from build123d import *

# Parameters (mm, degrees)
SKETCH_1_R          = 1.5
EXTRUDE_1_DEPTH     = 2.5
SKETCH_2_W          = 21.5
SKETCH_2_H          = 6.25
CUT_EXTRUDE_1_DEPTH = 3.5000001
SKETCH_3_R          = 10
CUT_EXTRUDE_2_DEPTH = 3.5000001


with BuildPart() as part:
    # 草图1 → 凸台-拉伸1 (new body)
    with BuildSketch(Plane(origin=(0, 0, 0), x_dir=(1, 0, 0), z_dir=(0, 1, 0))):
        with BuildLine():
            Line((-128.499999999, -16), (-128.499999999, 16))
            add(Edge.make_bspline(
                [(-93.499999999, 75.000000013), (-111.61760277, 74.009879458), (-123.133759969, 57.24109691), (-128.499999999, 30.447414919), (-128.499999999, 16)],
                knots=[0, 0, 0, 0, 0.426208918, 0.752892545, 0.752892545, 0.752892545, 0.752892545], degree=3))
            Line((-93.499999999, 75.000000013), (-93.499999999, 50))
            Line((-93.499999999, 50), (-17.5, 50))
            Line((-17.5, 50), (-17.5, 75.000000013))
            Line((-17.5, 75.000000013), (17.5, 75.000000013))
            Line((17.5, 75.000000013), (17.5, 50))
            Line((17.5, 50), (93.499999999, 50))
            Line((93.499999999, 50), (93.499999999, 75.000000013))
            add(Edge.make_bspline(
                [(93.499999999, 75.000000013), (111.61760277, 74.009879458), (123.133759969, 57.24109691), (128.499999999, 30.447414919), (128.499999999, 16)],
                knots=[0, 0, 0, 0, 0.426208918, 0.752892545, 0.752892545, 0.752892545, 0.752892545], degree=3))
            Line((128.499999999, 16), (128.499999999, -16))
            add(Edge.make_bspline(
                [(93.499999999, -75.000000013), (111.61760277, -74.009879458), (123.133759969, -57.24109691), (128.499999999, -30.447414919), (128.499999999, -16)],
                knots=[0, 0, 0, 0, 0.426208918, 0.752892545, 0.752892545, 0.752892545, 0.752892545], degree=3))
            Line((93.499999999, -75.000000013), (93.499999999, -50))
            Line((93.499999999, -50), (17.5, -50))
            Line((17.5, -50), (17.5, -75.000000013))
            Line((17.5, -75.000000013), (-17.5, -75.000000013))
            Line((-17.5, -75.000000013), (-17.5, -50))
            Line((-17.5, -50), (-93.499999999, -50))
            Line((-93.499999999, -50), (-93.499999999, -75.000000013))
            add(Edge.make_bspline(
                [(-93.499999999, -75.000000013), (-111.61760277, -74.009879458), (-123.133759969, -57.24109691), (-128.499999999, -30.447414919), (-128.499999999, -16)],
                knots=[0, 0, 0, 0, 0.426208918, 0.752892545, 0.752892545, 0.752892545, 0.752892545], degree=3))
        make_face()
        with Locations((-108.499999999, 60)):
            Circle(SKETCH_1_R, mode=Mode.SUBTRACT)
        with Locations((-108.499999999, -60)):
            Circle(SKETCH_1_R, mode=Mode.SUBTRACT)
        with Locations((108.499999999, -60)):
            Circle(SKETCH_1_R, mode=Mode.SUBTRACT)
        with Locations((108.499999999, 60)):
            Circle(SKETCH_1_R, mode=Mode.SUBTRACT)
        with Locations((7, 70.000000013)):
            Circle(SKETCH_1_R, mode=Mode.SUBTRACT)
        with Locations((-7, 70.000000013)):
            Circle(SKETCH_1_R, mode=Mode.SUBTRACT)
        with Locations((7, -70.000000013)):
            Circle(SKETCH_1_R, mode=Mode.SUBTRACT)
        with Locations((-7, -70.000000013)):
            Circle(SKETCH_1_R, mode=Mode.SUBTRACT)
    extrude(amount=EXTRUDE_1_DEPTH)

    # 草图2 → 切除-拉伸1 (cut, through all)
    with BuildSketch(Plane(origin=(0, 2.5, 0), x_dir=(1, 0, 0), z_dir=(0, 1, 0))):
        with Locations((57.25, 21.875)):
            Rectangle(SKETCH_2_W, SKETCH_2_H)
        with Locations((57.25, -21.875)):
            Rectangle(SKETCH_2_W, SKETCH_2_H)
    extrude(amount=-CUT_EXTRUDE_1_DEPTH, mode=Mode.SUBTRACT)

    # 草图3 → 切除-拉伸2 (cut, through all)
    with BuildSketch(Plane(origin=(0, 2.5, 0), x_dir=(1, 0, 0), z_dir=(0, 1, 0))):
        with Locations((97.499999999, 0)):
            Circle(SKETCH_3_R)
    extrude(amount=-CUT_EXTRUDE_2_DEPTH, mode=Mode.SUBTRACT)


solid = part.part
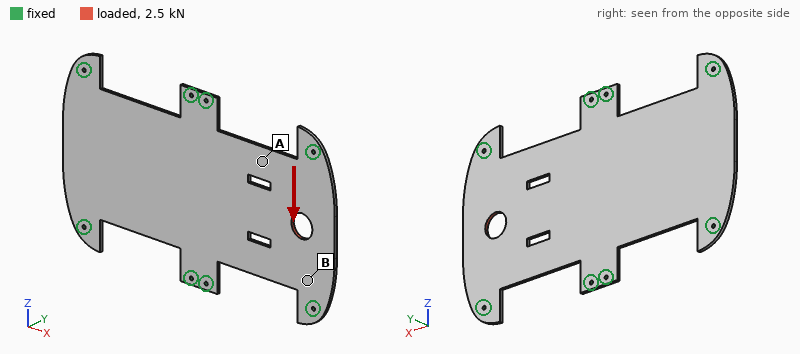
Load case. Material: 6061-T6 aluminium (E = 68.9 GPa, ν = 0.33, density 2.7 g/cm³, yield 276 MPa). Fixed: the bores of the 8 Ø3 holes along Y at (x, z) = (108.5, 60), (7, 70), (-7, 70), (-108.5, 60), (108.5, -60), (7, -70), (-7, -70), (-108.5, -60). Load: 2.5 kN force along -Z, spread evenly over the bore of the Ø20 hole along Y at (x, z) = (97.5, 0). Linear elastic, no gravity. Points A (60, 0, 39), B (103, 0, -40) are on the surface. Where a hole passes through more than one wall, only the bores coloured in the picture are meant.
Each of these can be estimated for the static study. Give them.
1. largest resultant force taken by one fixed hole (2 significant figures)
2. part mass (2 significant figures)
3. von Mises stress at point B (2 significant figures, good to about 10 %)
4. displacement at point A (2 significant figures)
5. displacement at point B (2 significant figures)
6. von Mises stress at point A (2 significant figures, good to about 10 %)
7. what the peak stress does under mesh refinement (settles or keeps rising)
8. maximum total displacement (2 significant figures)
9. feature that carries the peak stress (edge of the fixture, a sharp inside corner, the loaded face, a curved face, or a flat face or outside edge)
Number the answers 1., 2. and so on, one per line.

1. 1.1 kN
2. 190 g
3. 16 MPa
4. 8.4 µm
5. 7.2 µm
6. 3.9 MPa
7. keeps rising
8. 15 µm
9. edge of the fixture
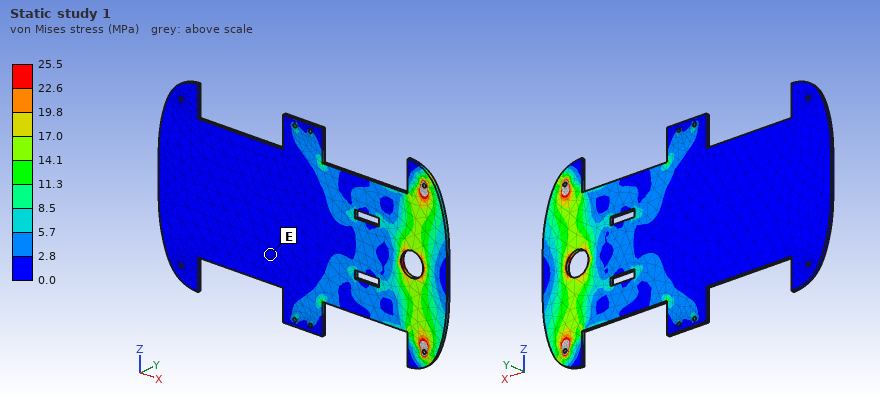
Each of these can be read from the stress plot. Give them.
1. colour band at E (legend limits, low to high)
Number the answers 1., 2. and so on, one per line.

1. 0.0 to 2.8 MPa
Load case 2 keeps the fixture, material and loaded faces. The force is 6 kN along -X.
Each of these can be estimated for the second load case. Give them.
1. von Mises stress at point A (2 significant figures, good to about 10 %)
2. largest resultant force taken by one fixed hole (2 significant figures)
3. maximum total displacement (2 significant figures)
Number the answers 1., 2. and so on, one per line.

1. 16 MPa
2. 1.3 kN
3. 74 µm
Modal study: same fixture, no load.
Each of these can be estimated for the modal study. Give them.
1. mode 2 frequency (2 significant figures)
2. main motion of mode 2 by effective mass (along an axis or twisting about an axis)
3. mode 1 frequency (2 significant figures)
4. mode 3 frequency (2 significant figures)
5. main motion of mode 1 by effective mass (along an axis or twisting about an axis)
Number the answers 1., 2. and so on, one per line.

1. 630 Hz
2. twisting about Z
3. 520 Hz
4. 880 Hz
5. along Y
